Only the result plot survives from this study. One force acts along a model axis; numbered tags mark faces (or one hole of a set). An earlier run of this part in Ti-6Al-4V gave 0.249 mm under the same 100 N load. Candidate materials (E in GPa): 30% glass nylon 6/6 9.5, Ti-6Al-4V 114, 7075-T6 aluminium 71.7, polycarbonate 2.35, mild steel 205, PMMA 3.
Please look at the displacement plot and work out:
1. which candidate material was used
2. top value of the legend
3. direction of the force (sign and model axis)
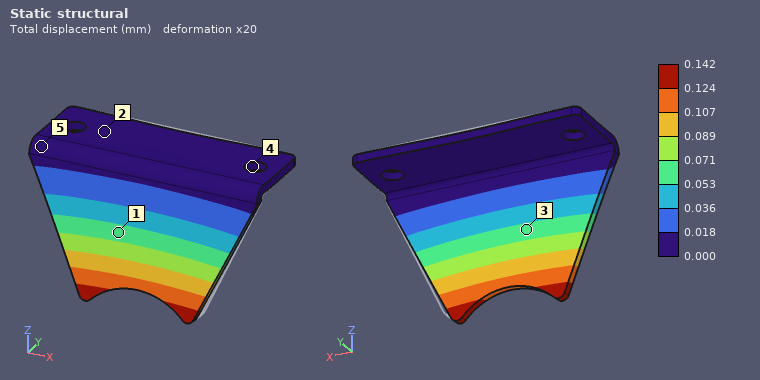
mild steel
0.142 mm
-Y
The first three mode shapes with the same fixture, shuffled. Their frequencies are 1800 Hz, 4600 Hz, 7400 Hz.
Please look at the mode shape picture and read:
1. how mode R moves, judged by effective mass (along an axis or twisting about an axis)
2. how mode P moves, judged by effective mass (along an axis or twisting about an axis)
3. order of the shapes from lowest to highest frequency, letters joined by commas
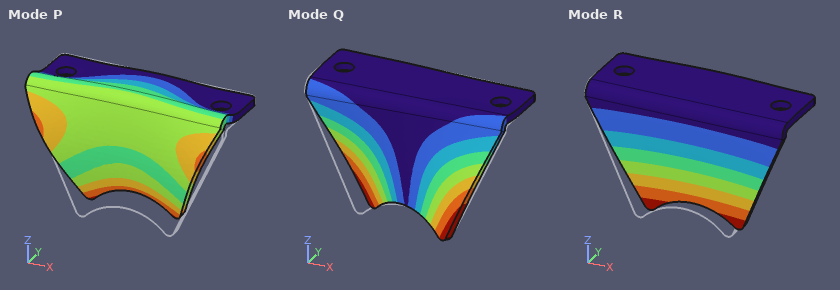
along Y
along Z
R, Q, P
